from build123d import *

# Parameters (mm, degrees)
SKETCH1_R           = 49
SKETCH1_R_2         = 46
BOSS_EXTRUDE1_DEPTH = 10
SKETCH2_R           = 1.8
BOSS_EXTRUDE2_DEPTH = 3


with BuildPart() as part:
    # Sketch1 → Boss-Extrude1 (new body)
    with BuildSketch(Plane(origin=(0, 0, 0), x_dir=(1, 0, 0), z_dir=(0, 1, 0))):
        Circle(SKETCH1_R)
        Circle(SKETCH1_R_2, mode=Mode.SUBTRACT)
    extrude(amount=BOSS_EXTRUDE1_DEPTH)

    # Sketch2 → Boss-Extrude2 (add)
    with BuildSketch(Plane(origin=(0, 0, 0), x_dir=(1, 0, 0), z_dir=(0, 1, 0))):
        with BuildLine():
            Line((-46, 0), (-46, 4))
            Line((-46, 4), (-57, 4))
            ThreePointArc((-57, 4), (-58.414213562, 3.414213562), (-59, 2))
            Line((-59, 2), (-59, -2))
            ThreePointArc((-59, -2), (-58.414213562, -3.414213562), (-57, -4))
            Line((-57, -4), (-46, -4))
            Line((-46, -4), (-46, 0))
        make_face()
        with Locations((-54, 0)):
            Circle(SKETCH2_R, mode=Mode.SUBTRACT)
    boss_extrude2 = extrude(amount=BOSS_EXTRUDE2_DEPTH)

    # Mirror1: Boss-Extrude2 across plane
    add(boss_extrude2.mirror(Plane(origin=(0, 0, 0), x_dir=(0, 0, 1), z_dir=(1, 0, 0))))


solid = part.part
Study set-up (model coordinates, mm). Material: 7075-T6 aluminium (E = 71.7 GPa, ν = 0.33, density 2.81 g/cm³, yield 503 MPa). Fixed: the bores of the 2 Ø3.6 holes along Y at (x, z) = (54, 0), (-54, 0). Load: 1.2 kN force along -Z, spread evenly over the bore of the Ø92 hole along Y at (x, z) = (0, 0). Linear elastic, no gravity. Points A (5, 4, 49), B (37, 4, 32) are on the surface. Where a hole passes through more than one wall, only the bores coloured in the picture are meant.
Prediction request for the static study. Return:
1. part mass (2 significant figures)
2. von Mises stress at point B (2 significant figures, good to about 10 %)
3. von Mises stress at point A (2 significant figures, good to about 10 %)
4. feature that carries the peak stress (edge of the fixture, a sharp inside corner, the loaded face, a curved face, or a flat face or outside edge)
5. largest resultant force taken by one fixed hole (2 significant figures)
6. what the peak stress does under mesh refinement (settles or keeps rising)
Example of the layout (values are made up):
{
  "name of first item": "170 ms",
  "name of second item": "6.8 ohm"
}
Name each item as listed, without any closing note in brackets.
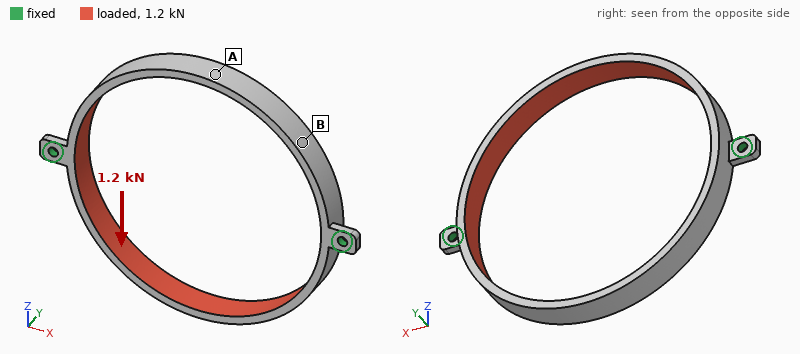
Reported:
{
  "part mass": "26 g",
  "von Mises stress at point B": "17 MPa",
  "von Mises stress at point A": "27 MPa",
  "feature that carries the peak stress": "edge of the fixture",
  "largest resultant force taken by one fixed hole": "600 N",
  "what the peak stress does under mesh refinement": "keeps rising"
}
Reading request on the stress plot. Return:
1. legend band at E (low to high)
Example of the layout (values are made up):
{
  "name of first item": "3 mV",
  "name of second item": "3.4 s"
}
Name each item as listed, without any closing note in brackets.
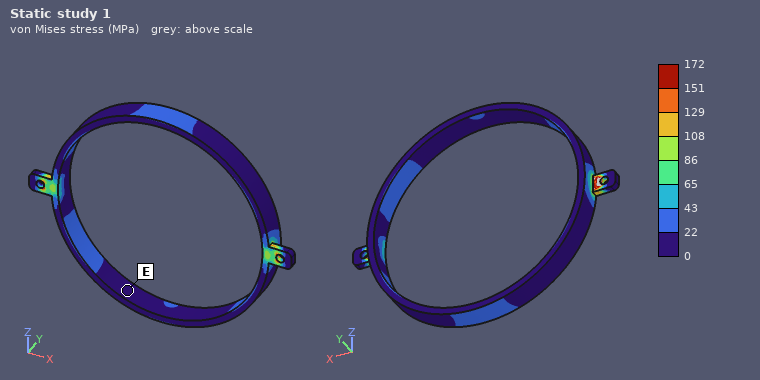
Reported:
{
  "legend band at E": "0 to 22 MPa"
}
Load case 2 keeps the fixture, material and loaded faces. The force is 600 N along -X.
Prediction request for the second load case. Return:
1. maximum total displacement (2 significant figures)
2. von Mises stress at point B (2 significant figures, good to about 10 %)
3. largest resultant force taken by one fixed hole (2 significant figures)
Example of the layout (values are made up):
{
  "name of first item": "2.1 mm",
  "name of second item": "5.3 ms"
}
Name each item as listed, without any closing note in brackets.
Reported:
{
  "maximum total displacement": "0.34 mm",
  "von Mises stress at point B": "45 MPa",
  "largest resultant force taken by one fixed hole": "300 N"
}
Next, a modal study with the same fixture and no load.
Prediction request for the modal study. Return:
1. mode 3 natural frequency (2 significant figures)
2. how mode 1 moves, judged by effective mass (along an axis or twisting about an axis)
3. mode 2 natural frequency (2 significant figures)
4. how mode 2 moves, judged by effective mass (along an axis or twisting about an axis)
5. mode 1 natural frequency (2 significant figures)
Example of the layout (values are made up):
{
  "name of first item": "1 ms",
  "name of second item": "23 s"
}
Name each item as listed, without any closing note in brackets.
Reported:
{
  "mode 3 natural frequency": "1300 Hz",
  "how mode 1 moves, judged by effective mass": "twisting about X",
  "mode 2 natural frequency": "1200 Hz",
  "how mode 2 moves, judged by effective mass": "along Y",
  "mode 1 natural frequency": "720 Hz"
}
